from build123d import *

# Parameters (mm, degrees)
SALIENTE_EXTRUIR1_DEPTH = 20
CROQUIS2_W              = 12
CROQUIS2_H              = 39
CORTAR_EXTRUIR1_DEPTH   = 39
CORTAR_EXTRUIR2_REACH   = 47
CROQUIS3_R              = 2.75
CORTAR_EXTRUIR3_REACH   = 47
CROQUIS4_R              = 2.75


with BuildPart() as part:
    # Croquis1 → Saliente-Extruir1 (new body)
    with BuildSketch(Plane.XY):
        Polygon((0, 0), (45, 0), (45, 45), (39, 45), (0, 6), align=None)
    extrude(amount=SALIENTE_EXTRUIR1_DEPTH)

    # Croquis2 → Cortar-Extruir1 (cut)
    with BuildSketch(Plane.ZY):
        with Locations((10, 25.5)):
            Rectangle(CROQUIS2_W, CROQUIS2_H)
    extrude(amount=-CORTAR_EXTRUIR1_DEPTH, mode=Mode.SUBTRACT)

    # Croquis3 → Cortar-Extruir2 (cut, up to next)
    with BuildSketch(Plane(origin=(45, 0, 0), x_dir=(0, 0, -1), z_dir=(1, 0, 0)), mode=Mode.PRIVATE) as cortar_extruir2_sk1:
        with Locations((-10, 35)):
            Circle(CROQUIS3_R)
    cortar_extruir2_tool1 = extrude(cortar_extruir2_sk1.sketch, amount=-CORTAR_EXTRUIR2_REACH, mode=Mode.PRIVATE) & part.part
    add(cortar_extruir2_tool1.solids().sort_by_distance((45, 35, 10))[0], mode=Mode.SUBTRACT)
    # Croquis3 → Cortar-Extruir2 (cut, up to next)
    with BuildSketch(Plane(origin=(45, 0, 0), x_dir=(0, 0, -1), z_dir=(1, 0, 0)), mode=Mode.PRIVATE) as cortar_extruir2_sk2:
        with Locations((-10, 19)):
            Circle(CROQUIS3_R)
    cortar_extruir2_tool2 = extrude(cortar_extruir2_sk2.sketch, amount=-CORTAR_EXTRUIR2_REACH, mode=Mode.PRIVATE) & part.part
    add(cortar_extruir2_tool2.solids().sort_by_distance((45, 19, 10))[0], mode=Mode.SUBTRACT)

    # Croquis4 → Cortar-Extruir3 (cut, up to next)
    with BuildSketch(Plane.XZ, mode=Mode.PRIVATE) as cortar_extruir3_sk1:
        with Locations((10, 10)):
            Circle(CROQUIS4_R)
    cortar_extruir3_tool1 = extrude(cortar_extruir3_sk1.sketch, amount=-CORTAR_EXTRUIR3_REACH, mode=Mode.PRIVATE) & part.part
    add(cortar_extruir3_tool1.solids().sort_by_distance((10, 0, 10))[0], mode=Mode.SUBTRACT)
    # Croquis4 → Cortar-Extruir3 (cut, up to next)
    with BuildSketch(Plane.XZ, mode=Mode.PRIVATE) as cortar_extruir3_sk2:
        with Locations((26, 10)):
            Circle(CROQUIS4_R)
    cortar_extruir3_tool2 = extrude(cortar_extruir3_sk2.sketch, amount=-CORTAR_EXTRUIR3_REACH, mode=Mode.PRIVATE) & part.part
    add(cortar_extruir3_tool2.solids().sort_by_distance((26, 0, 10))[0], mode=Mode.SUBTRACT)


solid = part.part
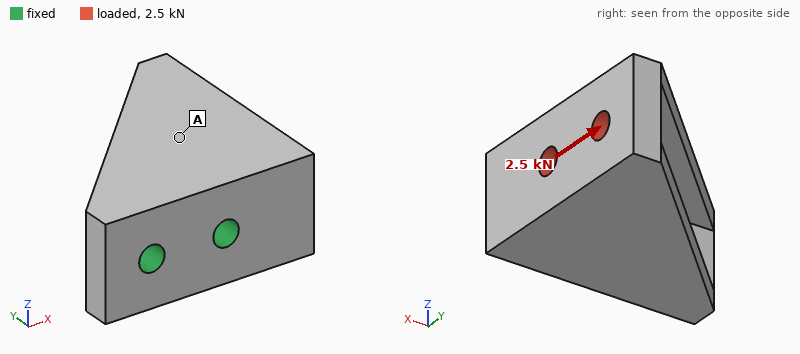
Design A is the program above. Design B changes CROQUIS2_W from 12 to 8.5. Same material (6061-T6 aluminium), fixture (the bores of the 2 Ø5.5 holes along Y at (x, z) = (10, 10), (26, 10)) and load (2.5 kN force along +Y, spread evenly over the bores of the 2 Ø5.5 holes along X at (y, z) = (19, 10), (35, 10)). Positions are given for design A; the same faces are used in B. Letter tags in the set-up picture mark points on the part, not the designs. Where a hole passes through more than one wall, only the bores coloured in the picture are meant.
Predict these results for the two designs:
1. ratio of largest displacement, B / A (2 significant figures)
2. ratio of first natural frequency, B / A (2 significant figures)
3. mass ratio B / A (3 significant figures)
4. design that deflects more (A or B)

0.79
1.1
1.17
A
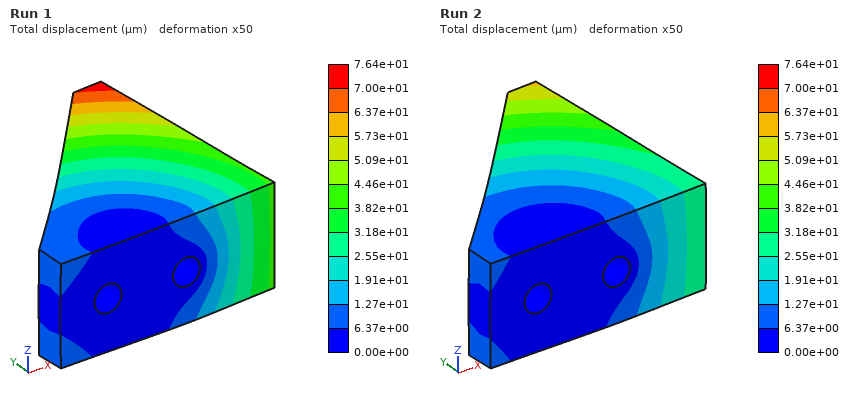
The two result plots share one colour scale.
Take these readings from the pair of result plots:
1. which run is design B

Run 2
